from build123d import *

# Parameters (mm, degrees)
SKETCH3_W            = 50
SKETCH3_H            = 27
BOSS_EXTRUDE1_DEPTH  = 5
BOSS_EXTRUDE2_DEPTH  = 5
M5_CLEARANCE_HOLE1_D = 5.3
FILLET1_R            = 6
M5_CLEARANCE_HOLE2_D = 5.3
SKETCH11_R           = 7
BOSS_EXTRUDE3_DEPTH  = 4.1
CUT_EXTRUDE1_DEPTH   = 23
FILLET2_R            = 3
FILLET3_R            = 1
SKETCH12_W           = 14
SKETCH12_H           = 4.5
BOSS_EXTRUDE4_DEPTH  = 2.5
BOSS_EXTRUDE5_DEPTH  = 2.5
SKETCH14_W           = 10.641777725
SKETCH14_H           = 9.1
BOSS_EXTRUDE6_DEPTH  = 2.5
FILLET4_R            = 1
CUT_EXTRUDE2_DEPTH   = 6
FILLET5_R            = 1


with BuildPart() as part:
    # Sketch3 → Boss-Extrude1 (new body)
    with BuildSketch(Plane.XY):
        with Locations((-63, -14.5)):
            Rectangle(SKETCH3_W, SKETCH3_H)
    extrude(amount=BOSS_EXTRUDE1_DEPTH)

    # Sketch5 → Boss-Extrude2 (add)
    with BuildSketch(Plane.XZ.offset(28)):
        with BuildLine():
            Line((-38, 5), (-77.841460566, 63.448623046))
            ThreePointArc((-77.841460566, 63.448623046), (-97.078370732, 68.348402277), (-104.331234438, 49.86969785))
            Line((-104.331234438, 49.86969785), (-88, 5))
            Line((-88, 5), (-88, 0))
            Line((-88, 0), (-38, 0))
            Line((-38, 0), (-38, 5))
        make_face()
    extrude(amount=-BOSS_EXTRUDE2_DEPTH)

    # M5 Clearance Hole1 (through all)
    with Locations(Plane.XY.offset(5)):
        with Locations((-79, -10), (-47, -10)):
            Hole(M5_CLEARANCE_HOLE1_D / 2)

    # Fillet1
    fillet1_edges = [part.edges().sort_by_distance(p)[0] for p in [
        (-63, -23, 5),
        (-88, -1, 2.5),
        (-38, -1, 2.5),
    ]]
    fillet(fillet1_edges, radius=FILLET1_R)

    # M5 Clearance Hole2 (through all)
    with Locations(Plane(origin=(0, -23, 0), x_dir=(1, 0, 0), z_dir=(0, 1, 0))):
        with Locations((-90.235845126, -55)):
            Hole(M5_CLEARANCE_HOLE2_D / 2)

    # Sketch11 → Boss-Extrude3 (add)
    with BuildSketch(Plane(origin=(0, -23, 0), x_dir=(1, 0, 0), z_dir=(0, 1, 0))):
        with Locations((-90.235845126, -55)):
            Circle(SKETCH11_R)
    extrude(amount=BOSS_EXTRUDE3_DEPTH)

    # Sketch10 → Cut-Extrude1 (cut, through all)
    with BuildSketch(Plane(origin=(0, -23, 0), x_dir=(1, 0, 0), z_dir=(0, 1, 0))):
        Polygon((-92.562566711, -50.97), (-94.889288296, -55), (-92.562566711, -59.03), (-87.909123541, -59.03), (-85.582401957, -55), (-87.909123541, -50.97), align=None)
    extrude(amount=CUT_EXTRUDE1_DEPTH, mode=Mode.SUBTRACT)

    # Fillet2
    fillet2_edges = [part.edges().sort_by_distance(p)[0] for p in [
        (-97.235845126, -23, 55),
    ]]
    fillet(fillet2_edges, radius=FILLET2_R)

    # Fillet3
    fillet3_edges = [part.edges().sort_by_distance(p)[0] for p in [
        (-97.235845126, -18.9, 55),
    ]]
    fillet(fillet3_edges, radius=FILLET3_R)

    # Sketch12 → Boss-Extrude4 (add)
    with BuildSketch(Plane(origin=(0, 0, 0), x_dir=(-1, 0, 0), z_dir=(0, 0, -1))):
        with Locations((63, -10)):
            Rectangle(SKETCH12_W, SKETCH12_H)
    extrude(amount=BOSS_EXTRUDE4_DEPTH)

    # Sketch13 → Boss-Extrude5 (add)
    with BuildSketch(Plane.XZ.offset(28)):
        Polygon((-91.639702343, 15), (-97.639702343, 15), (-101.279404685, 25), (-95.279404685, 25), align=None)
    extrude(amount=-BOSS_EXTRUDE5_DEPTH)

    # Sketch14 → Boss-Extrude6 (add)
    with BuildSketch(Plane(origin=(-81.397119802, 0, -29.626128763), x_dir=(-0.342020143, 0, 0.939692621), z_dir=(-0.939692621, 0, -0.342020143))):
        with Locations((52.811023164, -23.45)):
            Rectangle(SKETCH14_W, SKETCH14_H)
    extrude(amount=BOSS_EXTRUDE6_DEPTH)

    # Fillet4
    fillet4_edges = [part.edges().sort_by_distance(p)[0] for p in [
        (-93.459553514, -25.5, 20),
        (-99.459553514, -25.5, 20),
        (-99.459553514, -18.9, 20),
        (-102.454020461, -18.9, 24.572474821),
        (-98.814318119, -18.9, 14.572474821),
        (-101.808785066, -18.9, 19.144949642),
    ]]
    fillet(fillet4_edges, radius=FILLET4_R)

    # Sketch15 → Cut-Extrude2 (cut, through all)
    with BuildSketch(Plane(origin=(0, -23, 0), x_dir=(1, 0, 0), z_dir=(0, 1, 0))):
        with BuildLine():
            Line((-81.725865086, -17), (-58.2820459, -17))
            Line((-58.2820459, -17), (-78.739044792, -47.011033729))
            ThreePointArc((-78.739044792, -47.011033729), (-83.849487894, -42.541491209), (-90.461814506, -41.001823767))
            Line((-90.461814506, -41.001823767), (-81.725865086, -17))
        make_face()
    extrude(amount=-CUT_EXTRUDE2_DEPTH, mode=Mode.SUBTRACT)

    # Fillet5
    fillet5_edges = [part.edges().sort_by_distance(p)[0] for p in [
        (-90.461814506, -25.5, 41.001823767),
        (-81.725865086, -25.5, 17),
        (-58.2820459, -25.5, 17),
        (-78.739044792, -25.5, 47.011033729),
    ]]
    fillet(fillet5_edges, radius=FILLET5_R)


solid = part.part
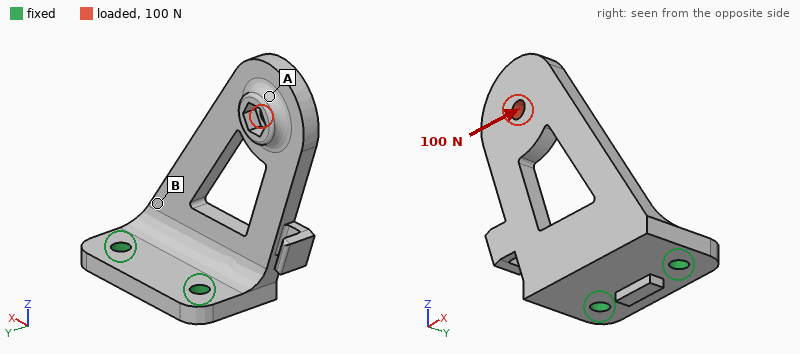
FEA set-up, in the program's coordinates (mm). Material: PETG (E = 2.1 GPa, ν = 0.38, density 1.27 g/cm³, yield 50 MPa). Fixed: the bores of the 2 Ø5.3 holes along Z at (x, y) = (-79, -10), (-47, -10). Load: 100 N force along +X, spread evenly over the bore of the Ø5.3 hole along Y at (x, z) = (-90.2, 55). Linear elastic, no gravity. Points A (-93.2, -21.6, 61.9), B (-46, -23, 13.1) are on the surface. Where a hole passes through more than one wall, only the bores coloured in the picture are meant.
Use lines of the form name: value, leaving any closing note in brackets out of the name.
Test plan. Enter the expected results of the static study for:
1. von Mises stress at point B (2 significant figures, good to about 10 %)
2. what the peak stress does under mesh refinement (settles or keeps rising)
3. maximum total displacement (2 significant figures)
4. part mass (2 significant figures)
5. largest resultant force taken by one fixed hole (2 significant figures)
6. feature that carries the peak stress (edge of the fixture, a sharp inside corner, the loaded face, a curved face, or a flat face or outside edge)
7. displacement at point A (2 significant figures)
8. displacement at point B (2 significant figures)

von Mises stress at point B: 8.1 MPa
what the peak stress does under mesh refinement: keeps rising
maximum total displacement: 1.1 mm
part mass: 22 g
largest resultant force taken by one fixed hole: 160 N
feature that carries the peak stress: edge of the fixture
displacement at point A: 1.0 mm
displacement at point B: 0.22 mm
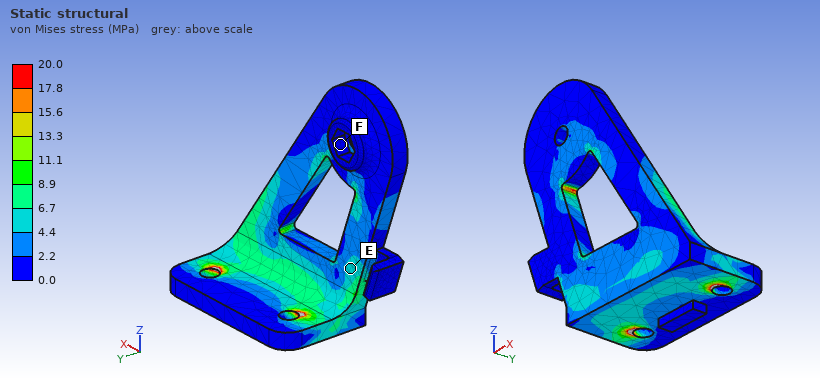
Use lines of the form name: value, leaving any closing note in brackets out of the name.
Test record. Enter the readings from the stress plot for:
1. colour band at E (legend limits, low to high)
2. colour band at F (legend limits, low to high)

colour band at E: 4.4 to 6.7 MPa
colour band at F: 0.0 to 2.2 MPa
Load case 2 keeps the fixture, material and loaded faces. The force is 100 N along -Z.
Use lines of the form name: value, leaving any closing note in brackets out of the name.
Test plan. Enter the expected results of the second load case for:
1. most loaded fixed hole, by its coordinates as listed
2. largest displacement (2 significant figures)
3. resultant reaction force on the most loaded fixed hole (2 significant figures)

most loaded fixed hole, by its coordinates as listed: (-79, -10)
largest displacement: 1.1 mm
resultant reaction force on the most loaded fixed hole: 130 N
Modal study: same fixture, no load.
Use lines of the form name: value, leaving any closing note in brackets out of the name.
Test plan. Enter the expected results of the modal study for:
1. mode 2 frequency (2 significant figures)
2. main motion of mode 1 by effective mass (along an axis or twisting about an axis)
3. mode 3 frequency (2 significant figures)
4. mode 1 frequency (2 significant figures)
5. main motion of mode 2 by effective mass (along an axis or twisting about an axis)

mode 2 frequency: 590 Hz
main motion of mode 1 by effective mass: along Y
mode 3 frequency: 830 Hz
mode 1 frequency: 190 Hz
main motion of mode 2 by effective mass: along X
